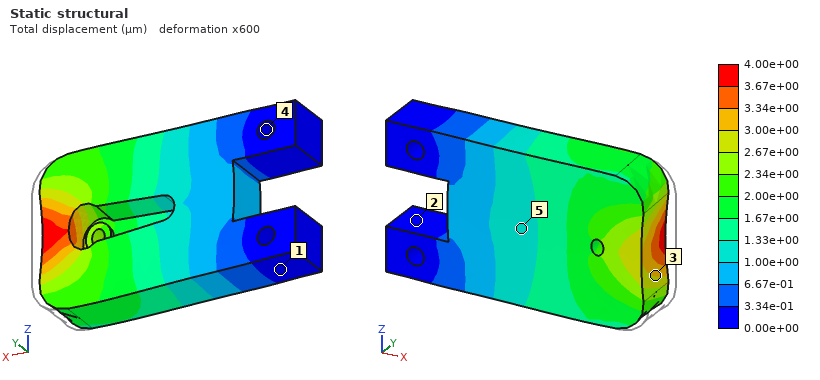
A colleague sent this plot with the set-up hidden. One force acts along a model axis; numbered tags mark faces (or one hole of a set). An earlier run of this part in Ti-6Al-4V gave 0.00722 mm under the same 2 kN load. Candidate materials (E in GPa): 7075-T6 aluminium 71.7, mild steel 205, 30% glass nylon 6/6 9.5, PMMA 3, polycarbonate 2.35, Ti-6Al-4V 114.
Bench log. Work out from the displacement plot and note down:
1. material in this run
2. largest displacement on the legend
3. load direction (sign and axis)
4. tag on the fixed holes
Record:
mild steel
4.00e+00 µm
-X
4
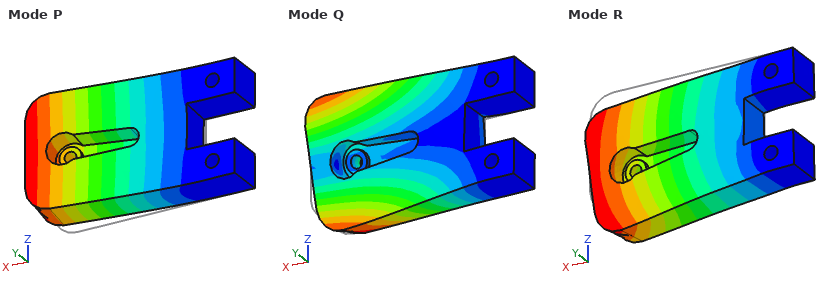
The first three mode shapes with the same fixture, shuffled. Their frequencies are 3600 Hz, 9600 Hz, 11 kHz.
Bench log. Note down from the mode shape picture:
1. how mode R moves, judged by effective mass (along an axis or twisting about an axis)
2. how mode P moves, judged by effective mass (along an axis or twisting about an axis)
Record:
along Z
along Y
